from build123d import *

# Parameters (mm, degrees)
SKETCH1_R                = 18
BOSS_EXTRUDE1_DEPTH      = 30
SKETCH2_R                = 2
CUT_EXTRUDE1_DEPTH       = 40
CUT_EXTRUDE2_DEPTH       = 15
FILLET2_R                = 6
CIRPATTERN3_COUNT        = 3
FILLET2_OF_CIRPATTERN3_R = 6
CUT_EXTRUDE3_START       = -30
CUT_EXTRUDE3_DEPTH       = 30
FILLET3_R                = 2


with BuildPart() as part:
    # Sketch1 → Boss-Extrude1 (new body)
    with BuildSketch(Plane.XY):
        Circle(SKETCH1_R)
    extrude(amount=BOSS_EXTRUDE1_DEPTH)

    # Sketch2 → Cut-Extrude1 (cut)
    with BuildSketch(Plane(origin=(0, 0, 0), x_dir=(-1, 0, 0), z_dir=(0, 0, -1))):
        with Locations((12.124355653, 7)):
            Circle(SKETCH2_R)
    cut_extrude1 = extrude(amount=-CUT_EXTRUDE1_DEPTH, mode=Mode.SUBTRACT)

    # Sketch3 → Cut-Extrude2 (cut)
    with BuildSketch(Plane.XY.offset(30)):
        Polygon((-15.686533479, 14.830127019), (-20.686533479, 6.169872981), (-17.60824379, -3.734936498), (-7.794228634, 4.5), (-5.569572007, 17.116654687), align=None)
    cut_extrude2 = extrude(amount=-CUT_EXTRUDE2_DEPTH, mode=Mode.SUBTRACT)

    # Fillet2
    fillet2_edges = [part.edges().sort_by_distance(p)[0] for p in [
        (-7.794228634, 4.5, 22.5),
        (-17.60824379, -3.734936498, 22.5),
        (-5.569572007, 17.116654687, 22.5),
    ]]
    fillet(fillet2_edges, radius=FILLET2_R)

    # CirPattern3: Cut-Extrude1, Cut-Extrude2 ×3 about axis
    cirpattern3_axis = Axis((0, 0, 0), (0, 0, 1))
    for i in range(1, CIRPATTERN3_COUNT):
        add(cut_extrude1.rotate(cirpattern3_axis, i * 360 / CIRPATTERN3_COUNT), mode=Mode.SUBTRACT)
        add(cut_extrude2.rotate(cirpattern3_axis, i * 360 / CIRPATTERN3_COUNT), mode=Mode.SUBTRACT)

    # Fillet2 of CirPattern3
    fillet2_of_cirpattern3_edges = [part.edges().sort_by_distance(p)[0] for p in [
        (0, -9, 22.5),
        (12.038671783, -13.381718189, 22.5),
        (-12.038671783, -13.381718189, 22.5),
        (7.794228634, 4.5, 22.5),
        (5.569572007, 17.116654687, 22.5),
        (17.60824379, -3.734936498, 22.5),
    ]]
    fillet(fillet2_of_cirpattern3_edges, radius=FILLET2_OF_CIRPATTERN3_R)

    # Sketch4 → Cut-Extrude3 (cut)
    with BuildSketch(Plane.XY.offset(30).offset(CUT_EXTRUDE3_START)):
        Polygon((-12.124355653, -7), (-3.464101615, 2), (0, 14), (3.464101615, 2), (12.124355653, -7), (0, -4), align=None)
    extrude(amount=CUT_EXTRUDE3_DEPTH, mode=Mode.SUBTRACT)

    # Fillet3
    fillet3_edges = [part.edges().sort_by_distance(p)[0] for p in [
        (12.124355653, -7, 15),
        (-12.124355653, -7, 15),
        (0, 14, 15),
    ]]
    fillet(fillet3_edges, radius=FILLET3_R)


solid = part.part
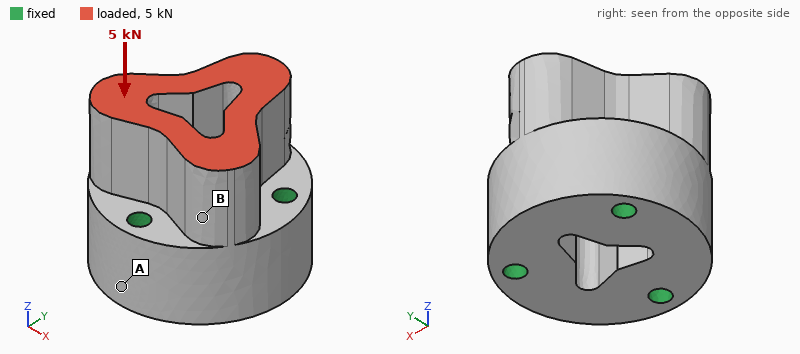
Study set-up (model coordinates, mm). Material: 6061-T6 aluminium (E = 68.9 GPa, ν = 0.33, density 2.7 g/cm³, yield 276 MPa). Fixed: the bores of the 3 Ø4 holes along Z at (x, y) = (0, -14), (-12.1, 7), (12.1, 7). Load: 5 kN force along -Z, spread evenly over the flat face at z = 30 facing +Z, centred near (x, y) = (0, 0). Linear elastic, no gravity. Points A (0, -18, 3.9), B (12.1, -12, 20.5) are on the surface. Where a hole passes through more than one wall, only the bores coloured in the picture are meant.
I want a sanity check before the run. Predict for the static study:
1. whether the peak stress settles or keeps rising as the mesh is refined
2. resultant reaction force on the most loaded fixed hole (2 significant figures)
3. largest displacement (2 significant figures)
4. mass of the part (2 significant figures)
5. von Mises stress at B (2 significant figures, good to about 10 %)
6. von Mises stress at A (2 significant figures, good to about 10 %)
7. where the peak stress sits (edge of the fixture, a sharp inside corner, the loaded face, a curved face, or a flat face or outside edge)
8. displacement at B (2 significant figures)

keeps rising
1.7 kN
4.9 µm
55 g
9.6 MPa
3.4 MPa
edge of the fixture
3.4 µm
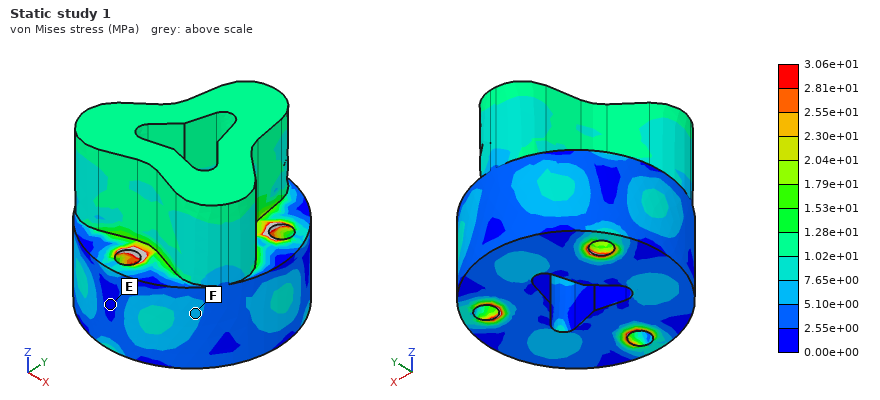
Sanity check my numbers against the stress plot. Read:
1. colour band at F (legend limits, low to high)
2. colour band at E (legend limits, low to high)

5.10e+00 to 7.65e+00 MPa
0.00e+00 to 2.55e+00 MPa
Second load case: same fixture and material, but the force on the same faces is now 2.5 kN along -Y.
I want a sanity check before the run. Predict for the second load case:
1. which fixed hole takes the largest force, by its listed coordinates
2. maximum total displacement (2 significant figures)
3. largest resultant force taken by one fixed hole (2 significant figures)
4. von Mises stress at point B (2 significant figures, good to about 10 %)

(0, -14)
20 µm
1.9 kN
19 MPa
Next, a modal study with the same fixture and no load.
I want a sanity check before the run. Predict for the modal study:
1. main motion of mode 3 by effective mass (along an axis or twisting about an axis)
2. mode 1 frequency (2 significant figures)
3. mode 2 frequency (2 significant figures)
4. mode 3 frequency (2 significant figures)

twisting about Z
21 kHz
21 kHz
33 kHz
